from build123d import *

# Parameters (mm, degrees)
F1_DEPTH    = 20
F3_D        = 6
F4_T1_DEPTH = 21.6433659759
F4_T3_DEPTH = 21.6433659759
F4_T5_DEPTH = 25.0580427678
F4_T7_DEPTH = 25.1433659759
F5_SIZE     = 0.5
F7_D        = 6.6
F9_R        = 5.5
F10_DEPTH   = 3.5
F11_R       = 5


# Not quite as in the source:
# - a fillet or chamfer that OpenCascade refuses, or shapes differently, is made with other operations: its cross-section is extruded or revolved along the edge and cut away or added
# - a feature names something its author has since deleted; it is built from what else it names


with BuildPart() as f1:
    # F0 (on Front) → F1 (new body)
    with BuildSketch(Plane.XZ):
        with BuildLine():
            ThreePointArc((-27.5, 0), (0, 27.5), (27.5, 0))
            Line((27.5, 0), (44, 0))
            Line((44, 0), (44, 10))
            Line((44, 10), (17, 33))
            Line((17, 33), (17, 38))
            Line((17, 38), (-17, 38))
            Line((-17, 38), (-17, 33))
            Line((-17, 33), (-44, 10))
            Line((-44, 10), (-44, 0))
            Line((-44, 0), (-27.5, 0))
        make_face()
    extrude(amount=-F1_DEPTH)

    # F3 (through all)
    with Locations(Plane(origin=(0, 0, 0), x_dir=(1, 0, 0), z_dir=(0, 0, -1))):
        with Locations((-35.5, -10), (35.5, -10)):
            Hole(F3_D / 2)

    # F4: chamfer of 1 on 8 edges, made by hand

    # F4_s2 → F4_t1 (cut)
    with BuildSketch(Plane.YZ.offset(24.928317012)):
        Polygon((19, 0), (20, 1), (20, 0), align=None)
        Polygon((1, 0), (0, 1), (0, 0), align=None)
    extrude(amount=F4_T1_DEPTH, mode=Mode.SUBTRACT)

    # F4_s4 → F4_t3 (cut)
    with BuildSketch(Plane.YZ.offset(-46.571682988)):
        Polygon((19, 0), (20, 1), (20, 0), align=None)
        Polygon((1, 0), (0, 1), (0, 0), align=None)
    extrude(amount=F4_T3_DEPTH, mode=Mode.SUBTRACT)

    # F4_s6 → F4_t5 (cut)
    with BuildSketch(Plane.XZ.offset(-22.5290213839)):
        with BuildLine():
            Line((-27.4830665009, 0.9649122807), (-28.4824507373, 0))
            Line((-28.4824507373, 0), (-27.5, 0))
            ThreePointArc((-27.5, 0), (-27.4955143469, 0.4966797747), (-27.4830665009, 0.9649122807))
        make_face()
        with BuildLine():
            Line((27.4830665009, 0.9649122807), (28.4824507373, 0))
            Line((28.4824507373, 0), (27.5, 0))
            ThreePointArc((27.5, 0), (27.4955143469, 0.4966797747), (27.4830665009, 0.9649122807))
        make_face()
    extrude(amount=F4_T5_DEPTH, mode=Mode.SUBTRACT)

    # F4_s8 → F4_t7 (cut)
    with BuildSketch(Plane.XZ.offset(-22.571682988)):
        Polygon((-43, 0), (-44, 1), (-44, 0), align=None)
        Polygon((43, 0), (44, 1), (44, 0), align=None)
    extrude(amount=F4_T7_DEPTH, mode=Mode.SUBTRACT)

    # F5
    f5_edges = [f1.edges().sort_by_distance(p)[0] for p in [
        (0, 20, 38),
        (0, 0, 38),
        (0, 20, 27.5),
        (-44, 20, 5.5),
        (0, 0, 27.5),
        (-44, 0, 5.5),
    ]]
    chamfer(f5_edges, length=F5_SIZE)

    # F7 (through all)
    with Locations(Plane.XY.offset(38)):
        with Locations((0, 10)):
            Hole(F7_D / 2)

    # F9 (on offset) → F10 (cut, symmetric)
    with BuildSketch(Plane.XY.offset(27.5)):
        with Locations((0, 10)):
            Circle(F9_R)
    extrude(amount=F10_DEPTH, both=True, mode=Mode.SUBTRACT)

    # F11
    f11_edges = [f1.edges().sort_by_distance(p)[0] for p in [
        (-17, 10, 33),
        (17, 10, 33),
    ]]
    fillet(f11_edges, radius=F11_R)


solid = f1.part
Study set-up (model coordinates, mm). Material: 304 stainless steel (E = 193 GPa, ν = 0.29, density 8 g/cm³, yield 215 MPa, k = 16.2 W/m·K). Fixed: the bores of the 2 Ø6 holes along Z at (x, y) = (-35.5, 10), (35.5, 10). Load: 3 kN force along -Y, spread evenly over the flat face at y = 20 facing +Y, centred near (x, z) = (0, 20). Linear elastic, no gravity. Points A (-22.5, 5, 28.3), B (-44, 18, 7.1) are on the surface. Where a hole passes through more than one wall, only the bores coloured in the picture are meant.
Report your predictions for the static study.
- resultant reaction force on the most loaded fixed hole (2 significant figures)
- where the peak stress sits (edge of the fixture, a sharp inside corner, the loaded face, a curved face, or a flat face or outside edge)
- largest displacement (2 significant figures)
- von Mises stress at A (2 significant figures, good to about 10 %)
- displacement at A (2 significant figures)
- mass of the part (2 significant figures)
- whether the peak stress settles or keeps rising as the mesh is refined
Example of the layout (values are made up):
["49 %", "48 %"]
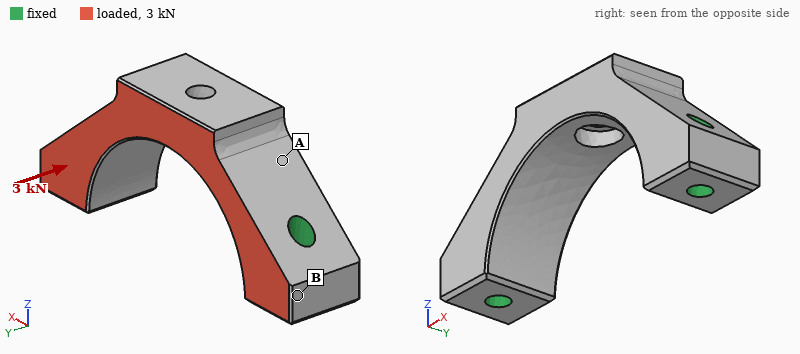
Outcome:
["1.5 kN", "edge of the fixture", "9.1 µm", "15 MPa", "4.4 µm", "190 g", "keeps rising"]
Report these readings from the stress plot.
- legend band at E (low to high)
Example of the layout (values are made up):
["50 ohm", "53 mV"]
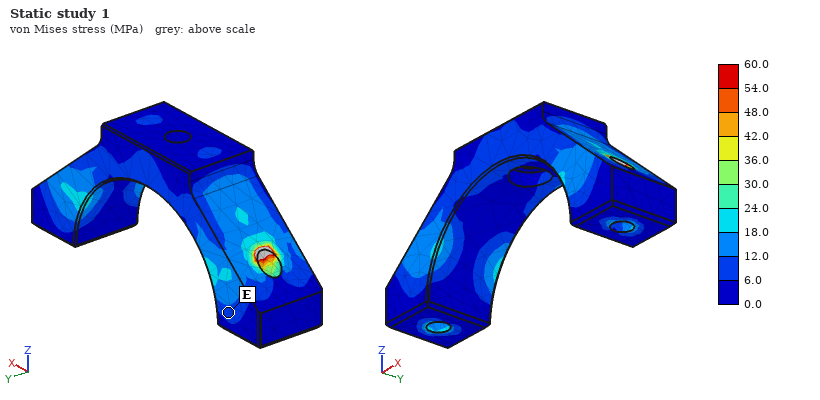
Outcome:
["6.0 to 12.0 MPa"]
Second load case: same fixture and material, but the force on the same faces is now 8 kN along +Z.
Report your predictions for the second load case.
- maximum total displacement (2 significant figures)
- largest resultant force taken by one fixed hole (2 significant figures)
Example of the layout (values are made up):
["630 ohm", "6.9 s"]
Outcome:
["20 µm", "4.3 kN"]
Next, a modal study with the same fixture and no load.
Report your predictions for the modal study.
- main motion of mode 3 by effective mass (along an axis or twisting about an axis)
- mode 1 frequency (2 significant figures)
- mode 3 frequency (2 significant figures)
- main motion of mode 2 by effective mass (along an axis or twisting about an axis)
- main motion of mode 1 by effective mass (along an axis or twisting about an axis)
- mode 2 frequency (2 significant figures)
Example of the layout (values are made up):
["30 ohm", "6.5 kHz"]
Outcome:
["along Z", "7900 Hz", "18 kHz", "along X", "along Y", "16 kHz"]
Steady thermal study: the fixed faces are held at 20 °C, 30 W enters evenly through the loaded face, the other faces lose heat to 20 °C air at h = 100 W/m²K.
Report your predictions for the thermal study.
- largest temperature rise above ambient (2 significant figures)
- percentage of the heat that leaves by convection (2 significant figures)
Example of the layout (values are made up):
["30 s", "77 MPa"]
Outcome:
["42 K", "33 %"]
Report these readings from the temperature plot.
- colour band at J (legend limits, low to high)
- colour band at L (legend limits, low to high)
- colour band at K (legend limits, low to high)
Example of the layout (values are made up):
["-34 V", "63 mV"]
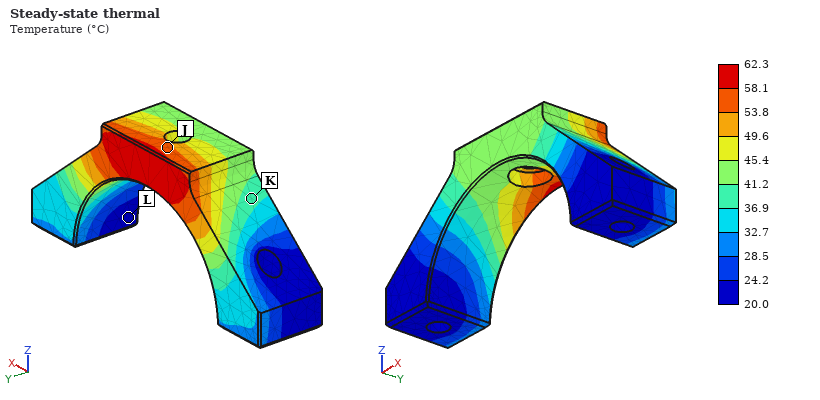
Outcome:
["53.8 to 58.1 °C", "20.0 to 24.2 °C", "36.9 to 41.2 °C"]
